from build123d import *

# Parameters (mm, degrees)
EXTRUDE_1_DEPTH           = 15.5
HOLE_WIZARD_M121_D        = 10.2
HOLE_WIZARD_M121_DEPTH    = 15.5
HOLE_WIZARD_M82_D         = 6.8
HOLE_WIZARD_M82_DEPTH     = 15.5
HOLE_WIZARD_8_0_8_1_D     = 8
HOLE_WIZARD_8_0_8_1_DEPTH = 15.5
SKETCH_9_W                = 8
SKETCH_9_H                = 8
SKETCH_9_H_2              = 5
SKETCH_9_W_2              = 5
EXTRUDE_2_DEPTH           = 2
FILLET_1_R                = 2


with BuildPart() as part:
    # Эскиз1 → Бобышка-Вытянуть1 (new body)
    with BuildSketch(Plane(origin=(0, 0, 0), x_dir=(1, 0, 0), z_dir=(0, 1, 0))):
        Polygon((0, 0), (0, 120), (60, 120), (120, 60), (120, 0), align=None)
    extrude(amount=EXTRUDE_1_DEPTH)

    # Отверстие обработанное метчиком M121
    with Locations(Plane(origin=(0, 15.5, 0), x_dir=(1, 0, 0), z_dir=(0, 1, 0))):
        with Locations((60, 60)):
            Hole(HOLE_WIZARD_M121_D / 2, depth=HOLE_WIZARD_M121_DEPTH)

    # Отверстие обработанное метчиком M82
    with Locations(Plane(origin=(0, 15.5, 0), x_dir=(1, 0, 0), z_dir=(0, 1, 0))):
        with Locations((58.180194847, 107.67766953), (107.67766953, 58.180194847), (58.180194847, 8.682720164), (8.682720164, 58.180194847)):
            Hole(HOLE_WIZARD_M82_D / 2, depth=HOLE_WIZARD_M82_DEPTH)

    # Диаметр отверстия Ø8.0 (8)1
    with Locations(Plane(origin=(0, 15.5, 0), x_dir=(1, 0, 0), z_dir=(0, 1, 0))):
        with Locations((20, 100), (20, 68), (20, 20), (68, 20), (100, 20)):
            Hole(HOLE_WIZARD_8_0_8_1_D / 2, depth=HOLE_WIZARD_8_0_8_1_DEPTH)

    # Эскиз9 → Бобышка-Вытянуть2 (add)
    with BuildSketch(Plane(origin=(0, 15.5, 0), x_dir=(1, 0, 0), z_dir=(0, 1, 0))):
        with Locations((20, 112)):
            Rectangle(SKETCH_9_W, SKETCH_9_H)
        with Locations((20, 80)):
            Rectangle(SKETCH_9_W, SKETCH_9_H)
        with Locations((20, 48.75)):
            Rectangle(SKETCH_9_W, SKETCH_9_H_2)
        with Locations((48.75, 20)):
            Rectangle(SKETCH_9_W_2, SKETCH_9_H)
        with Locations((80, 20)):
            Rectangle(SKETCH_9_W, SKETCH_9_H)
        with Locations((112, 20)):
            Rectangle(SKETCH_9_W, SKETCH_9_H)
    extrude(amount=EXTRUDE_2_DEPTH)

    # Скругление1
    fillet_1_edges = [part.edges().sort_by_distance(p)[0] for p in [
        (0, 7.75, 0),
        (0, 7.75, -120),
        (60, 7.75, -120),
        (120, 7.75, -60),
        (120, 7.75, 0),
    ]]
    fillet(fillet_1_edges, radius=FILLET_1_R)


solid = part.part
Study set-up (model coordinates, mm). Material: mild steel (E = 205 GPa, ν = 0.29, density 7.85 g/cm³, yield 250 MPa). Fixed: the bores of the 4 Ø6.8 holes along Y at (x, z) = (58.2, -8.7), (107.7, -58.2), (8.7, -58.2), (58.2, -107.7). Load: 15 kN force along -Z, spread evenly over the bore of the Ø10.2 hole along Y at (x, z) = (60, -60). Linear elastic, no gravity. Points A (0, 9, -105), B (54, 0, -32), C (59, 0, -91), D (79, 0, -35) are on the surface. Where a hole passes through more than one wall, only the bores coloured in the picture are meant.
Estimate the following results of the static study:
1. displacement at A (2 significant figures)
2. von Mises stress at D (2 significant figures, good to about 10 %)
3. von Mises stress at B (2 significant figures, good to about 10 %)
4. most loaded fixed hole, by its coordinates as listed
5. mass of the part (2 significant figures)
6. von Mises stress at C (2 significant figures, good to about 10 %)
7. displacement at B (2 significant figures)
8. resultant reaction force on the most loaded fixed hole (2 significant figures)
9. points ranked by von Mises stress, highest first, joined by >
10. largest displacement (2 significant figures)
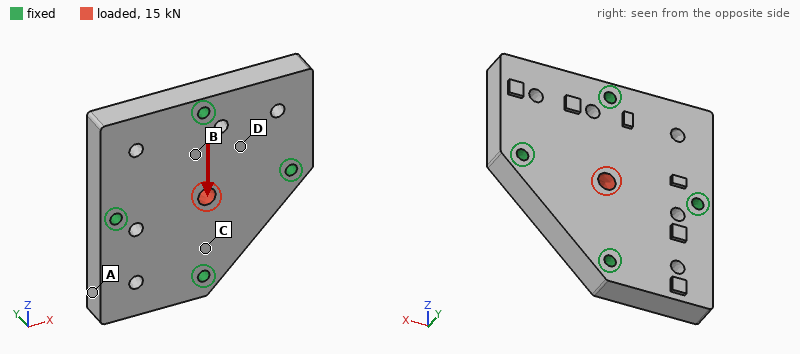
0.69 µm
7.0 MPa
14 MPa
(58.2, -107.7)
1.5 kg
17 MPa
1.6 µm
5.4 kN
C > B > D > A
3.9 µm
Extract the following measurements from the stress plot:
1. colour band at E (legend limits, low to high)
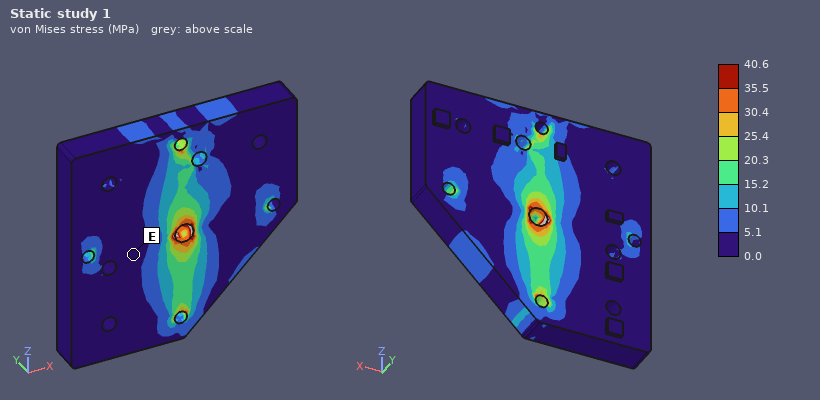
0.0 to 5.1 MPa
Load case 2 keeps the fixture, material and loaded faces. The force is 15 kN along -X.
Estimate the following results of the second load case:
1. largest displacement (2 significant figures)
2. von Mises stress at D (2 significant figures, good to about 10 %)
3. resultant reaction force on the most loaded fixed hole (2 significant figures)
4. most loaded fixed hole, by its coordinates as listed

3.9 µm
4.1 MPa
5.4 kN
(107.7, -58.2)
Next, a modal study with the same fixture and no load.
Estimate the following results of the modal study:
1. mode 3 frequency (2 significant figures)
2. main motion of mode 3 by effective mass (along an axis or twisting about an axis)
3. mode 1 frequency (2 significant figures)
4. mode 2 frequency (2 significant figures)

6600 Hz
along Y
6000 Hz
6100 Hz
